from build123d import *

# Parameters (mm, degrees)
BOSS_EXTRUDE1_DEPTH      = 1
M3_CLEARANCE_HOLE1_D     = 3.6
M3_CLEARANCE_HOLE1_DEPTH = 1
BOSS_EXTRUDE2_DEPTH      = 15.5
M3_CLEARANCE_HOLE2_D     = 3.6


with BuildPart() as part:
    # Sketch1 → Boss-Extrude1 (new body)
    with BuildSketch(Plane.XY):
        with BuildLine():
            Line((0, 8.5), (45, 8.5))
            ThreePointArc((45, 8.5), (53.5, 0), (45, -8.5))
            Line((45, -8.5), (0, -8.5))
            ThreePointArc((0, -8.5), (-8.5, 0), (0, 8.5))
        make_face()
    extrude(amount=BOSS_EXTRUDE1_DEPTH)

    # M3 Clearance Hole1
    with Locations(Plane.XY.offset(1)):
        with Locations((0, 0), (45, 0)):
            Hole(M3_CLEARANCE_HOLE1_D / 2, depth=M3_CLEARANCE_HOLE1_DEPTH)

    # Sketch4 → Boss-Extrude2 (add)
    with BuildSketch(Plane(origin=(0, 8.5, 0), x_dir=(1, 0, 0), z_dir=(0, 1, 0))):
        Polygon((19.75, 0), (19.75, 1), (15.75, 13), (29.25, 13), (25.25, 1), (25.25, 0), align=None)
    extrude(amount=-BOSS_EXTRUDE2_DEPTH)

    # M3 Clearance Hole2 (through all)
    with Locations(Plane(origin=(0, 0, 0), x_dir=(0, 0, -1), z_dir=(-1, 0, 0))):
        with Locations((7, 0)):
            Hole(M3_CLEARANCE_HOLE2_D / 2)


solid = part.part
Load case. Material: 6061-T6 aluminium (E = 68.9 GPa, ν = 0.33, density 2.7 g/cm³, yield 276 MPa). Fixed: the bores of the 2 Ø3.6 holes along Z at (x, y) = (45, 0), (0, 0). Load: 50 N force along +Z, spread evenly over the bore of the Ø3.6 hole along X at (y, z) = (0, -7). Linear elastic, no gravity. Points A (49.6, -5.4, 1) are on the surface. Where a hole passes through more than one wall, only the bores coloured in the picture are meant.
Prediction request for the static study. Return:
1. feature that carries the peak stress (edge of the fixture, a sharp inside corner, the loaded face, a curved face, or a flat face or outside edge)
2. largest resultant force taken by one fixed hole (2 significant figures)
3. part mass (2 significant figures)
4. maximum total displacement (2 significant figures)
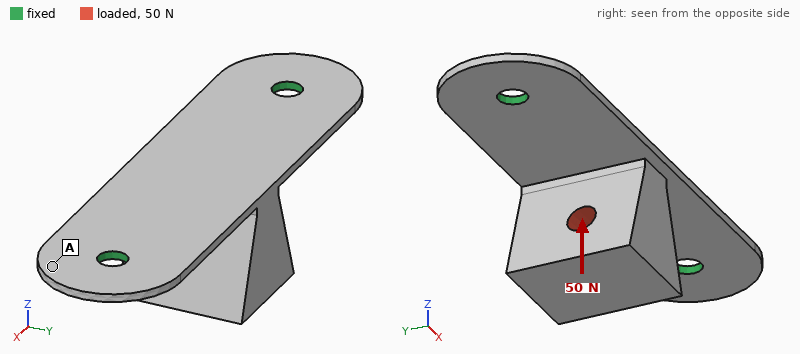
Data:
a flat face or outside edge
28 N
7.4 g
0.15 mm
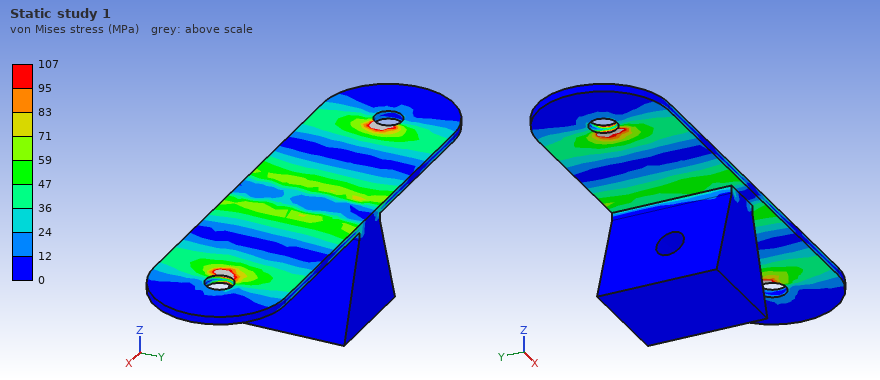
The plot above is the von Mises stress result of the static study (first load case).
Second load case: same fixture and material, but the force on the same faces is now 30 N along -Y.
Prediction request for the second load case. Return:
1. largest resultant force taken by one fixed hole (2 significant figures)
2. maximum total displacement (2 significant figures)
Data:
15 N
0.19 mm
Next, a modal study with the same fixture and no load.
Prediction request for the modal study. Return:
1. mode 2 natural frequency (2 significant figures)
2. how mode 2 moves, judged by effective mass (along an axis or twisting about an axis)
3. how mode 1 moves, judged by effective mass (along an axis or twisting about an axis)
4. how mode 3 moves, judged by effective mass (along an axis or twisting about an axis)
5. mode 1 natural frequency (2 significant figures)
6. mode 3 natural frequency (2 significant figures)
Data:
1200 Hz
along Z
along Y
along X
990 Hz
1800 Hz
